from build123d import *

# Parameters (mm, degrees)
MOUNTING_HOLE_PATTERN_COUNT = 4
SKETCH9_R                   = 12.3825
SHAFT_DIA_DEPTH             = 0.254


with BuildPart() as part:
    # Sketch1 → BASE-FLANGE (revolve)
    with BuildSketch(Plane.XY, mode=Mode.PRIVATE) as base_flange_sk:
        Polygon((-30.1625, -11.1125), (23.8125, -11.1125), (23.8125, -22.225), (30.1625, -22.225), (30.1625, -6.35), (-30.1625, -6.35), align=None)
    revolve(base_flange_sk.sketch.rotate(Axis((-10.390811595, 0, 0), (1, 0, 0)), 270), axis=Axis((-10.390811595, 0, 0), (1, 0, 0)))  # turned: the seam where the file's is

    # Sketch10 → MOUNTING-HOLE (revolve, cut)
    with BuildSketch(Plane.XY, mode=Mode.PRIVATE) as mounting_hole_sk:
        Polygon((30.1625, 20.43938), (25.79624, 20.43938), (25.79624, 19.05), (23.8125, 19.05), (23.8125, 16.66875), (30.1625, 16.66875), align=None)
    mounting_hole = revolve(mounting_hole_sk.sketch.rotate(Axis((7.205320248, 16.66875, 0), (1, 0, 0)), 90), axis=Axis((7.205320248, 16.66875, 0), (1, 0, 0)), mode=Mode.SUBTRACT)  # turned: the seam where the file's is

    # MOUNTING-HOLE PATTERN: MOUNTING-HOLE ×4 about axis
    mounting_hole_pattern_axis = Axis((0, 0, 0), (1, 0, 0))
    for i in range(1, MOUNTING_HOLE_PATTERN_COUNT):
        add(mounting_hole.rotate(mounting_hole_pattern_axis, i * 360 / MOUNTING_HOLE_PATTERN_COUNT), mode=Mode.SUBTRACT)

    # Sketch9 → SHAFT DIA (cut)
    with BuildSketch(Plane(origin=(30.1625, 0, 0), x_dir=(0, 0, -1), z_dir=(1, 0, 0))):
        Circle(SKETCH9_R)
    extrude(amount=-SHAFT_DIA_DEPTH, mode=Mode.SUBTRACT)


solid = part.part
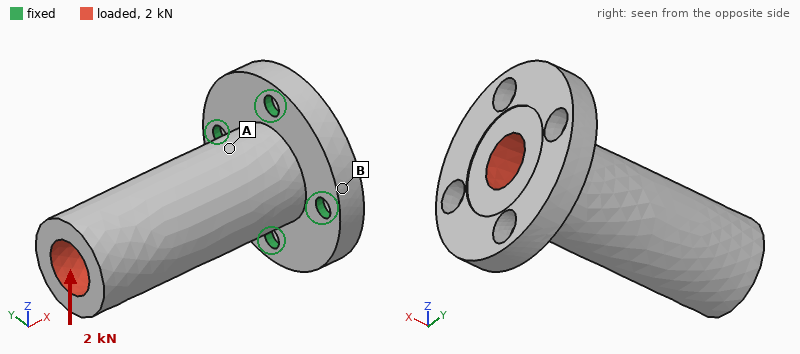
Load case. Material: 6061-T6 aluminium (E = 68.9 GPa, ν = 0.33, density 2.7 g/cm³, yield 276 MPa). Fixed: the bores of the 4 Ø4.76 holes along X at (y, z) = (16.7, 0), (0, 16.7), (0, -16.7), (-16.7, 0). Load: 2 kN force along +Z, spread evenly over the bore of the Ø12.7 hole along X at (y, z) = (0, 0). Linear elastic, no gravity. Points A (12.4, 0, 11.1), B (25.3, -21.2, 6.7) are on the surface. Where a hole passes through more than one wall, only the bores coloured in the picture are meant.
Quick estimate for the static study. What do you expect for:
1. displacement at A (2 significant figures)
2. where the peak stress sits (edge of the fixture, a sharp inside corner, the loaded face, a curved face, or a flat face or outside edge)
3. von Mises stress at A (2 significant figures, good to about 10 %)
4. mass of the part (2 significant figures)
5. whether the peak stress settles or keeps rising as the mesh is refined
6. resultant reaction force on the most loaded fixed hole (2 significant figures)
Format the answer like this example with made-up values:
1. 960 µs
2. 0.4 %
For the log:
1. 0.032 mm
2. edge of the fixture
3. 29 MPa
4. 60 g
5. keeps rising
6. 1.6 kN
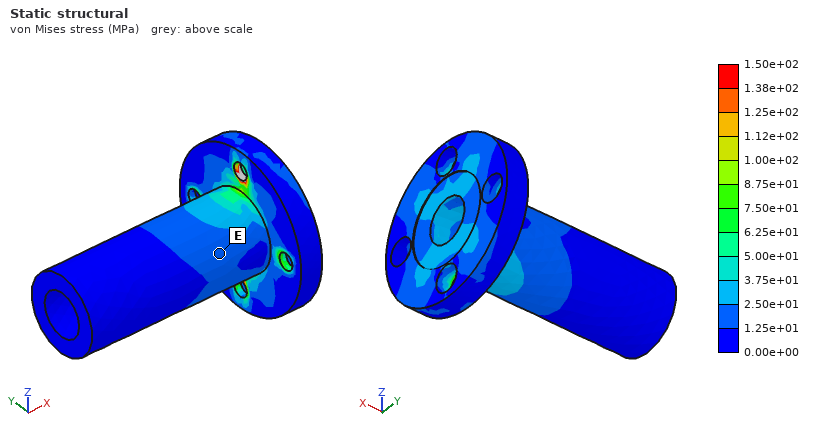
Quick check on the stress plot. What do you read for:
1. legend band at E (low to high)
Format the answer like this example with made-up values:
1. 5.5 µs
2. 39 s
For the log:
1. 1.25e+01 to 2.50e+01 MPa
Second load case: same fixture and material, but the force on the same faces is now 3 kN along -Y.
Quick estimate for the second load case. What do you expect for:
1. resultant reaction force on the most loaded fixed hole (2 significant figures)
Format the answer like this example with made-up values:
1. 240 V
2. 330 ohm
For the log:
1. 2.4 kN
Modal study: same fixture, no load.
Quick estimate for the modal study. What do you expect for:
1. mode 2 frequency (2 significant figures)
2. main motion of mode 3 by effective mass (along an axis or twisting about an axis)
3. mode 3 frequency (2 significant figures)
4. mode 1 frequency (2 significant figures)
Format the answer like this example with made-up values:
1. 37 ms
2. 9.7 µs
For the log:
1. 3700 Hz
2. along X
3. 13 kHz
4. 3700 Hz
